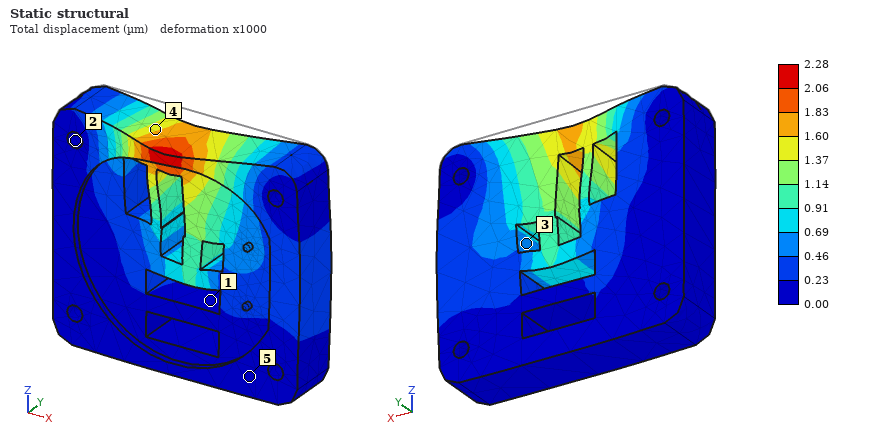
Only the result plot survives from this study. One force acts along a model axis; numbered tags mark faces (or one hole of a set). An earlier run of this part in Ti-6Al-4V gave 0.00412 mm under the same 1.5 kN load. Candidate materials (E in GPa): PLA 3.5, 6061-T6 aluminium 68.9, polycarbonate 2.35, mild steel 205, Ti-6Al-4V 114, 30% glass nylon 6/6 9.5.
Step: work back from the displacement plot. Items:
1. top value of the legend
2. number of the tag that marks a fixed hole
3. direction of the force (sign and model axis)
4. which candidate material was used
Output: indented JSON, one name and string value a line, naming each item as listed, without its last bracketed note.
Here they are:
{
  "top value of the legend": "2.28 µm",
  "number of the tag that marks a fixed hole": "2",
  "direction of the force": "-Z",
  "which candidate material was used": "mild steel"
}
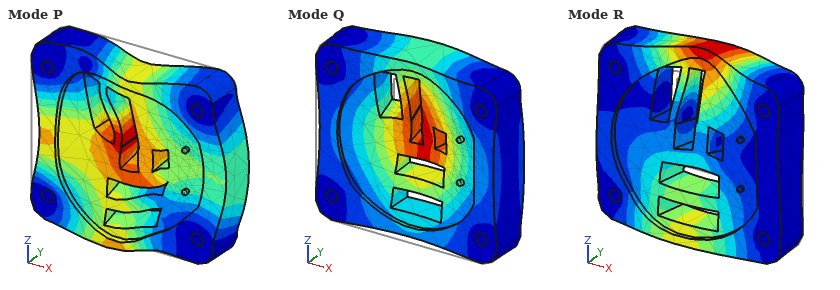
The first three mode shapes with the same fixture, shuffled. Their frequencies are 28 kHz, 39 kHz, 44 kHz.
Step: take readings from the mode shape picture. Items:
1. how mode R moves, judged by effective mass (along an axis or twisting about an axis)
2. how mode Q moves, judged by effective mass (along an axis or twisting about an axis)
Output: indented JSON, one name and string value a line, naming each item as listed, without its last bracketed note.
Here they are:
{
  "how mode R moves, judged by effective mass": "twisting about X",
  "how mode Q moves, judged by effective mass": "along Y"
}
